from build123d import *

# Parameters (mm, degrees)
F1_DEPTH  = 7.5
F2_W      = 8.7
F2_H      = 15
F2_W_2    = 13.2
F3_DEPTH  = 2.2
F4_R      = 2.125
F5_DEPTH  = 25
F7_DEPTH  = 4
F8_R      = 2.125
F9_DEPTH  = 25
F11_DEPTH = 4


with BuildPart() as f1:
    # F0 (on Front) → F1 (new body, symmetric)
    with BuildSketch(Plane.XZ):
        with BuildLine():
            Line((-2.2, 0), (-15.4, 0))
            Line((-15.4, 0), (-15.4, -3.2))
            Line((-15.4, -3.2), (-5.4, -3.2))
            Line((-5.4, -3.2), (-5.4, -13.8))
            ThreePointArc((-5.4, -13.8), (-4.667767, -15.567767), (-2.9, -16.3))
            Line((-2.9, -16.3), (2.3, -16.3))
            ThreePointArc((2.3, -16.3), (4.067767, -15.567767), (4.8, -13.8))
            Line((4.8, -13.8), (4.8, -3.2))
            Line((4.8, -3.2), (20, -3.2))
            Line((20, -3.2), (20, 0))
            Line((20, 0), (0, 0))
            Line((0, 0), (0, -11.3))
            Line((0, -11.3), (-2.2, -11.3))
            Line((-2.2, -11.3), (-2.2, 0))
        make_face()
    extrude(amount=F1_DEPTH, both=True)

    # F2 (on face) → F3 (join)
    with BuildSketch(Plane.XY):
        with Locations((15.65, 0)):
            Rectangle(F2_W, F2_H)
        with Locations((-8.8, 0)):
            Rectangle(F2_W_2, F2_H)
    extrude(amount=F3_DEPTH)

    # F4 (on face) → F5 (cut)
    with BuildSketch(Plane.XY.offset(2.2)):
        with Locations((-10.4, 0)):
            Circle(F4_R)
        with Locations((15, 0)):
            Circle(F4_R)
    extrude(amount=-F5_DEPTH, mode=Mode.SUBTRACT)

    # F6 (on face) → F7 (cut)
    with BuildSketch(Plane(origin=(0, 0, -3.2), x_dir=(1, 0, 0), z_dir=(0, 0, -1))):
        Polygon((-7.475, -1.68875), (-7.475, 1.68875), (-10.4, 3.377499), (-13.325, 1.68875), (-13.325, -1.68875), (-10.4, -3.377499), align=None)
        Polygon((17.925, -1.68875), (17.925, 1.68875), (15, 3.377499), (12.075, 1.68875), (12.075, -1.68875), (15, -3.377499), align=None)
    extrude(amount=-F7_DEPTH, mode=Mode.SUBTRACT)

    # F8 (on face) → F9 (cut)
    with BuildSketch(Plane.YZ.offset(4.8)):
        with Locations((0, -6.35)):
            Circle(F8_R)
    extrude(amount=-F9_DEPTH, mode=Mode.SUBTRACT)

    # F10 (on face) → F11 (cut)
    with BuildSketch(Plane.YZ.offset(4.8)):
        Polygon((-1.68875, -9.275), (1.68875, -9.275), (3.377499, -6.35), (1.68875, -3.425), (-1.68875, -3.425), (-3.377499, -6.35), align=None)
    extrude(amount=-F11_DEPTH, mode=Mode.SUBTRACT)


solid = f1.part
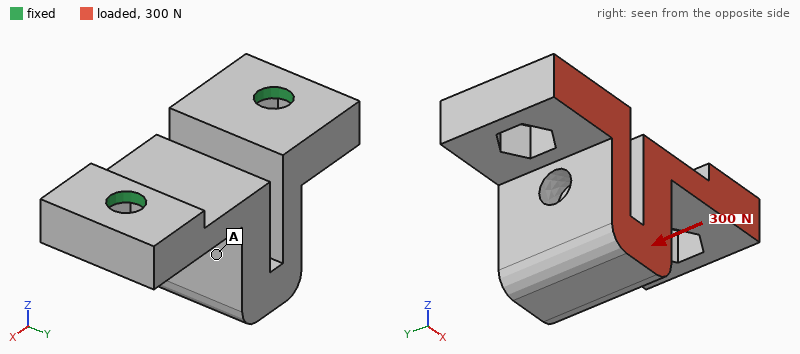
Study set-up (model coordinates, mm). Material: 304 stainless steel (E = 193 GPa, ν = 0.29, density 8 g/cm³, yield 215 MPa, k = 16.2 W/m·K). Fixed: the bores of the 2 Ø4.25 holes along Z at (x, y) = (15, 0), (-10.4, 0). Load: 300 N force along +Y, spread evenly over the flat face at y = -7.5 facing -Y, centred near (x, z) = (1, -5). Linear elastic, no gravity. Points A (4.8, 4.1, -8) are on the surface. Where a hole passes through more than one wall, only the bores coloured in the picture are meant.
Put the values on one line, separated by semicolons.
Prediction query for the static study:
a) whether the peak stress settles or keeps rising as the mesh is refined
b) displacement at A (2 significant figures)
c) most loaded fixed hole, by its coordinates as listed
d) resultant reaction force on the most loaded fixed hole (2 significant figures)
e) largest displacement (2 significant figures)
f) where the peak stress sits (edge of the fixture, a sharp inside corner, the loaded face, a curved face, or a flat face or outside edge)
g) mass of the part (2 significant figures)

keeps rising; 6.3 µm; (-10.4, 0); 160 N; 11 µm; edge of the fixture; 28 g
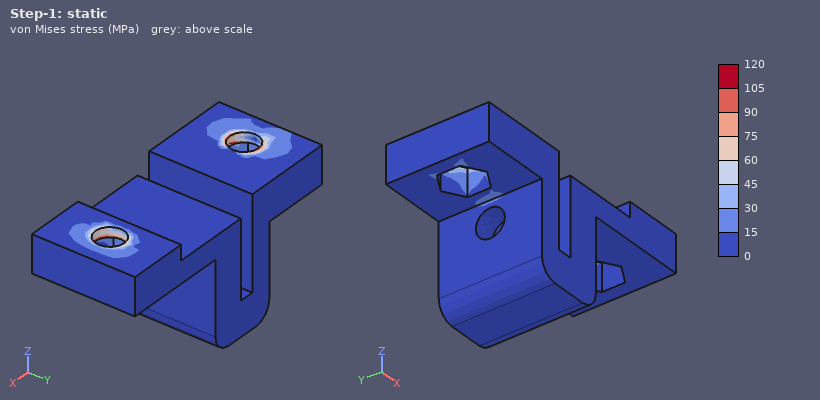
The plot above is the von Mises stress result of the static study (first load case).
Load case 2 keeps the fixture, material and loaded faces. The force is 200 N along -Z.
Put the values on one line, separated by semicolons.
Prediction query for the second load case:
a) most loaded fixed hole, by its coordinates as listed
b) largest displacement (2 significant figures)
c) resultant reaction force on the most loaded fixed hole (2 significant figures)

(-10.4, 0); 8.2 µm; 110 N
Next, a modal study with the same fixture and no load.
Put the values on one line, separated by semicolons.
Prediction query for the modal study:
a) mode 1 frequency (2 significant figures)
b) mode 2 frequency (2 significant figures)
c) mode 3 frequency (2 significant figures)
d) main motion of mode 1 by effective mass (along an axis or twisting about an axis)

5600 Hz; 11 kHz; 16 kHz; along Y
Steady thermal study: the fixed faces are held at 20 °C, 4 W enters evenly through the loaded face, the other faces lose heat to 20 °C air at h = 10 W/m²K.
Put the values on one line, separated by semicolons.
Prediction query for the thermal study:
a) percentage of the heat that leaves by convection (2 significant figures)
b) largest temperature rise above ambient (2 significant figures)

10 %; 32 K
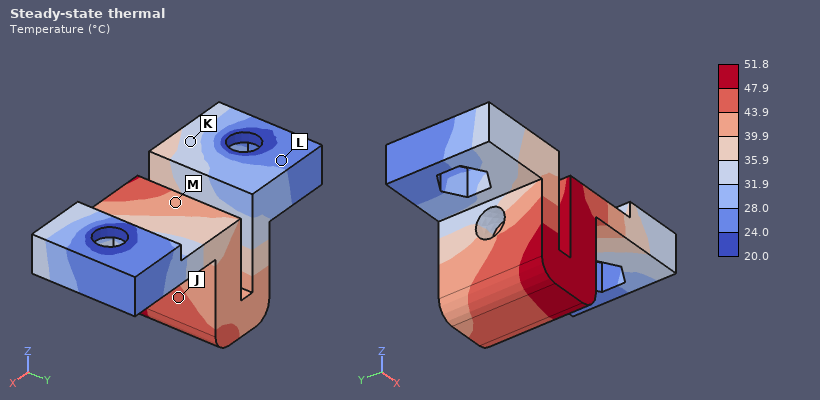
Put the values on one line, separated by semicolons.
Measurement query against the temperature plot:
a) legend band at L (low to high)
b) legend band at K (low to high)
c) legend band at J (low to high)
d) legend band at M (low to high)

24.0 to 28.0 °C; 31.9 to 35.9 °C; 43.9 to 47.9 °C; 39.9 to 43.9 °C
